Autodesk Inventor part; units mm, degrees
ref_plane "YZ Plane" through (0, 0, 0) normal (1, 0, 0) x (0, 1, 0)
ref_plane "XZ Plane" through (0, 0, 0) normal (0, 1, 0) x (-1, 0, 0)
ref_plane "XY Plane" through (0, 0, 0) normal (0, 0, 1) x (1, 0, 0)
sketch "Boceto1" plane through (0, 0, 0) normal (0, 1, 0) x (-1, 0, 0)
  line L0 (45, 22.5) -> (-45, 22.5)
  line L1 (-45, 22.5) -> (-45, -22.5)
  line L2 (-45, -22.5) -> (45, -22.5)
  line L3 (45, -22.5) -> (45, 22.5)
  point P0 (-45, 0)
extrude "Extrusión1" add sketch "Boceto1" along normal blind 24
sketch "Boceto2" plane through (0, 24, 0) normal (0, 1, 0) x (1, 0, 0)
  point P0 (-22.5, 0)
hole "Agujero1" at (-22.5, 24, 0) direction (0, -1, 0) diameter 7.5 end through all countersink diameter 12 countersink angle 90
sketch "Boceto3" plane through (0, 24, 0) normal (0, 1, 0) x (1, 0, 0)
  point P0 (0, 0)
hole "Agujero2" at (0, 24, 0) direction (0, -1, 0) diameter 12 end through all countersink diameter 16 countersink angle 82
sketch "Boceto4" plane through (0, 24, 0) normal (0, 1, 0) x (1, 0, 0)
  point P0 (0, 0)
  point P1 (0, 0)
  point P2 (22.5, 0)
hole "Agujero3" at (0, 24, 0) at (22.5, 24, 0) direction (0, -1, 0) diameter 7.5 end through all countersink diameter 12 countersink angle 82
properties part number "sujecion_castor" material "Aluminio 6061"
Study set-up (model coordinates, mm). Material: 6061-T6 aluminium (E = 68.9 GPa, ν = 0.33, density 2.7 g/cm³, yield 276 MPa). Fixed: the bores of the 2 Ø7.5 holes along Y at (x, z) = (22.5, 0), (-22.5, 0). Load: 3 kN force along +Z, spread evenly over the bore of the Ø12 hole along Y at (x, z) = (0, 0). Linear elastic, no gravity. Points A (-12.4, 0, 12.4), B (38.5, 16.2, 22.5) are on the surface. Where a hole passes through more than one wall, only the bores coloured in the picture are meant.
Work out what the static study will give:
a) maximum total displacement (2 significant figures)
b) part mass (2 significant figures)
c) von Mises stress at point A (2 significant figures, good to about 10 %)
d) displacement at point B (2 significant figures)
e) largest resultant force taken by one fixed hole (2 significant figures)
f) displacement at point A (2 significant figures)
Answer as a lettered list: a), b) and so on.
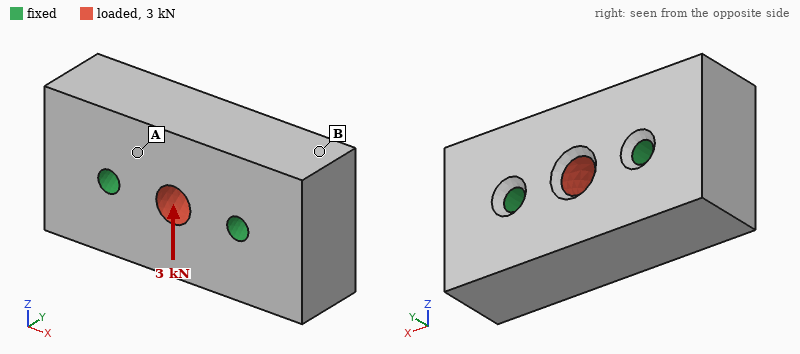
a) 1.9 µm
b) 250 g
c) 3.2 MPa
d) 0.60 µm
e) 1.5 kN
f) 0.97 µm
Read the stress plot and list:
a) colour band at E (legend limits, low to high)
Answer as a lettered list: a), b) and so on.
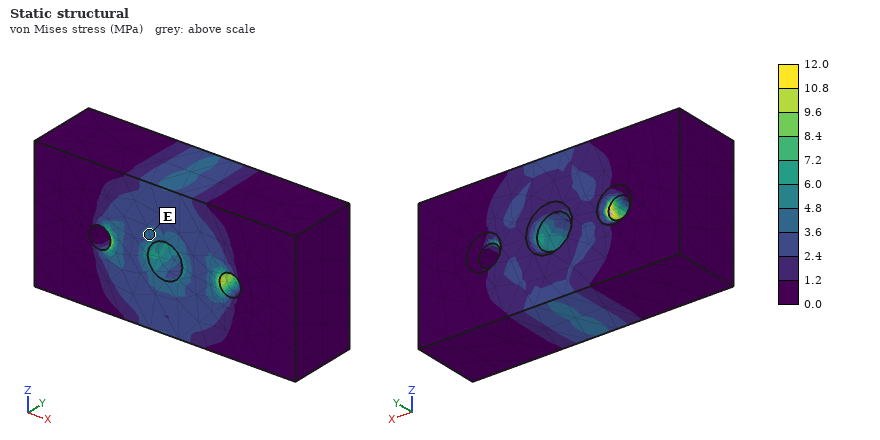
a) 3.6 to 4.8 MPa
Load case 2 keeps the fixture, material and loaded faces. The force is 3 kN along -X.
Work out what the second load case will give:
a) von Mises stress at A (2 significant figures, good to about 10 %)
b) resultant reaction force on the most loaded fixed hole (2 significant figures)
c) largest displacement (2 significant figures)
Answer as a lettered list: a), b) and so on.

a) 0.93 MPa
b) 1.5 kN
c) 0.97 µm
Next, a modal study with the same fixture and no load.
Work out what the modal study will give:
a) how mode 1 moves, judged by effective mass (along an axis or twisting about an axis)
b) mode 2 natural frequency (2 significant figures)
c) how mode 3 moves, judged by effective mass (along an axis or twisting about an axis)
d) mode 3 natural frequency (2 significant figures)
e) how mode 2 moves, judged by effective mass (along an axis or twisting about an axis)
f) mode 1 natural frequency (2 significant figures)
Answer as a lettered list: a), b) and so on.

a) twisting about X
b) 16 kHz
c) twisting about Z
d) 18 kHz
e) twisting about Y
f) 15 kHz
